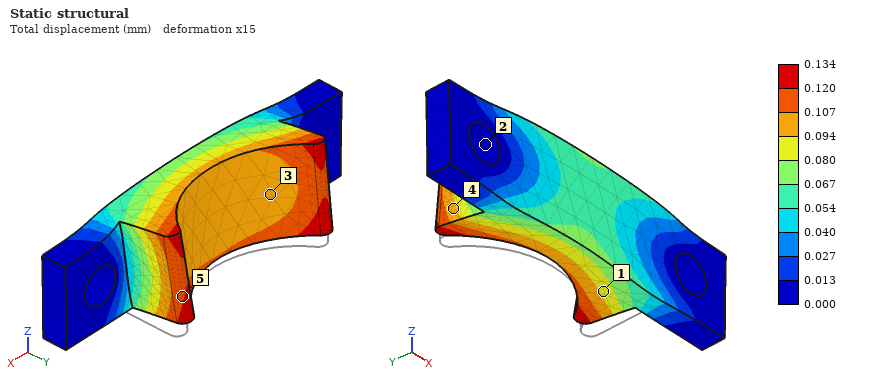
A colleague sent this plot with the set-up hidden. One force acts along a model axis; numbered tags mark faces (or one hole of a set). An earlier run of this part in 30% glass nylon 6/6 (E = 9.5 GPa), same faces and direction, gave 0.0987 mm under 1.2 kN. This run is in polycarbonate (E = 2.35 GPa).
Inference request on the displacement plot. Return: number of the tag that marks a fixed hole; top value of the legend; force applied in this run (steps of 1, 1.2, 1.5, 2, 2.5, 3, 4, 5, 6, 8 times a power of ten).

2
0.134 mm
400 N
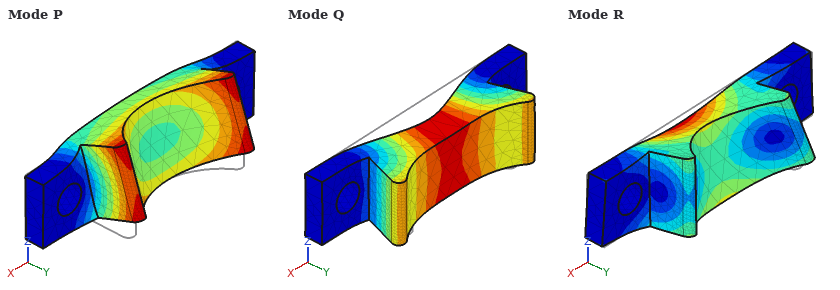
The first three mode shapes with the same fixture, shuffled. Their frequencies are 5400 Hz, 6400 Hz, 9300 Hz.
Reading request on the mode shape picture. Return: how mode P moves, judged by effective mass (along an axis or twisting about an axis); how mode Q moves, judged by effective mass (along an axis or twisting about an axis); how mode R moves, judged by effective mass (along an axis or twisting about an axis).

along Z
along Y
along Z
